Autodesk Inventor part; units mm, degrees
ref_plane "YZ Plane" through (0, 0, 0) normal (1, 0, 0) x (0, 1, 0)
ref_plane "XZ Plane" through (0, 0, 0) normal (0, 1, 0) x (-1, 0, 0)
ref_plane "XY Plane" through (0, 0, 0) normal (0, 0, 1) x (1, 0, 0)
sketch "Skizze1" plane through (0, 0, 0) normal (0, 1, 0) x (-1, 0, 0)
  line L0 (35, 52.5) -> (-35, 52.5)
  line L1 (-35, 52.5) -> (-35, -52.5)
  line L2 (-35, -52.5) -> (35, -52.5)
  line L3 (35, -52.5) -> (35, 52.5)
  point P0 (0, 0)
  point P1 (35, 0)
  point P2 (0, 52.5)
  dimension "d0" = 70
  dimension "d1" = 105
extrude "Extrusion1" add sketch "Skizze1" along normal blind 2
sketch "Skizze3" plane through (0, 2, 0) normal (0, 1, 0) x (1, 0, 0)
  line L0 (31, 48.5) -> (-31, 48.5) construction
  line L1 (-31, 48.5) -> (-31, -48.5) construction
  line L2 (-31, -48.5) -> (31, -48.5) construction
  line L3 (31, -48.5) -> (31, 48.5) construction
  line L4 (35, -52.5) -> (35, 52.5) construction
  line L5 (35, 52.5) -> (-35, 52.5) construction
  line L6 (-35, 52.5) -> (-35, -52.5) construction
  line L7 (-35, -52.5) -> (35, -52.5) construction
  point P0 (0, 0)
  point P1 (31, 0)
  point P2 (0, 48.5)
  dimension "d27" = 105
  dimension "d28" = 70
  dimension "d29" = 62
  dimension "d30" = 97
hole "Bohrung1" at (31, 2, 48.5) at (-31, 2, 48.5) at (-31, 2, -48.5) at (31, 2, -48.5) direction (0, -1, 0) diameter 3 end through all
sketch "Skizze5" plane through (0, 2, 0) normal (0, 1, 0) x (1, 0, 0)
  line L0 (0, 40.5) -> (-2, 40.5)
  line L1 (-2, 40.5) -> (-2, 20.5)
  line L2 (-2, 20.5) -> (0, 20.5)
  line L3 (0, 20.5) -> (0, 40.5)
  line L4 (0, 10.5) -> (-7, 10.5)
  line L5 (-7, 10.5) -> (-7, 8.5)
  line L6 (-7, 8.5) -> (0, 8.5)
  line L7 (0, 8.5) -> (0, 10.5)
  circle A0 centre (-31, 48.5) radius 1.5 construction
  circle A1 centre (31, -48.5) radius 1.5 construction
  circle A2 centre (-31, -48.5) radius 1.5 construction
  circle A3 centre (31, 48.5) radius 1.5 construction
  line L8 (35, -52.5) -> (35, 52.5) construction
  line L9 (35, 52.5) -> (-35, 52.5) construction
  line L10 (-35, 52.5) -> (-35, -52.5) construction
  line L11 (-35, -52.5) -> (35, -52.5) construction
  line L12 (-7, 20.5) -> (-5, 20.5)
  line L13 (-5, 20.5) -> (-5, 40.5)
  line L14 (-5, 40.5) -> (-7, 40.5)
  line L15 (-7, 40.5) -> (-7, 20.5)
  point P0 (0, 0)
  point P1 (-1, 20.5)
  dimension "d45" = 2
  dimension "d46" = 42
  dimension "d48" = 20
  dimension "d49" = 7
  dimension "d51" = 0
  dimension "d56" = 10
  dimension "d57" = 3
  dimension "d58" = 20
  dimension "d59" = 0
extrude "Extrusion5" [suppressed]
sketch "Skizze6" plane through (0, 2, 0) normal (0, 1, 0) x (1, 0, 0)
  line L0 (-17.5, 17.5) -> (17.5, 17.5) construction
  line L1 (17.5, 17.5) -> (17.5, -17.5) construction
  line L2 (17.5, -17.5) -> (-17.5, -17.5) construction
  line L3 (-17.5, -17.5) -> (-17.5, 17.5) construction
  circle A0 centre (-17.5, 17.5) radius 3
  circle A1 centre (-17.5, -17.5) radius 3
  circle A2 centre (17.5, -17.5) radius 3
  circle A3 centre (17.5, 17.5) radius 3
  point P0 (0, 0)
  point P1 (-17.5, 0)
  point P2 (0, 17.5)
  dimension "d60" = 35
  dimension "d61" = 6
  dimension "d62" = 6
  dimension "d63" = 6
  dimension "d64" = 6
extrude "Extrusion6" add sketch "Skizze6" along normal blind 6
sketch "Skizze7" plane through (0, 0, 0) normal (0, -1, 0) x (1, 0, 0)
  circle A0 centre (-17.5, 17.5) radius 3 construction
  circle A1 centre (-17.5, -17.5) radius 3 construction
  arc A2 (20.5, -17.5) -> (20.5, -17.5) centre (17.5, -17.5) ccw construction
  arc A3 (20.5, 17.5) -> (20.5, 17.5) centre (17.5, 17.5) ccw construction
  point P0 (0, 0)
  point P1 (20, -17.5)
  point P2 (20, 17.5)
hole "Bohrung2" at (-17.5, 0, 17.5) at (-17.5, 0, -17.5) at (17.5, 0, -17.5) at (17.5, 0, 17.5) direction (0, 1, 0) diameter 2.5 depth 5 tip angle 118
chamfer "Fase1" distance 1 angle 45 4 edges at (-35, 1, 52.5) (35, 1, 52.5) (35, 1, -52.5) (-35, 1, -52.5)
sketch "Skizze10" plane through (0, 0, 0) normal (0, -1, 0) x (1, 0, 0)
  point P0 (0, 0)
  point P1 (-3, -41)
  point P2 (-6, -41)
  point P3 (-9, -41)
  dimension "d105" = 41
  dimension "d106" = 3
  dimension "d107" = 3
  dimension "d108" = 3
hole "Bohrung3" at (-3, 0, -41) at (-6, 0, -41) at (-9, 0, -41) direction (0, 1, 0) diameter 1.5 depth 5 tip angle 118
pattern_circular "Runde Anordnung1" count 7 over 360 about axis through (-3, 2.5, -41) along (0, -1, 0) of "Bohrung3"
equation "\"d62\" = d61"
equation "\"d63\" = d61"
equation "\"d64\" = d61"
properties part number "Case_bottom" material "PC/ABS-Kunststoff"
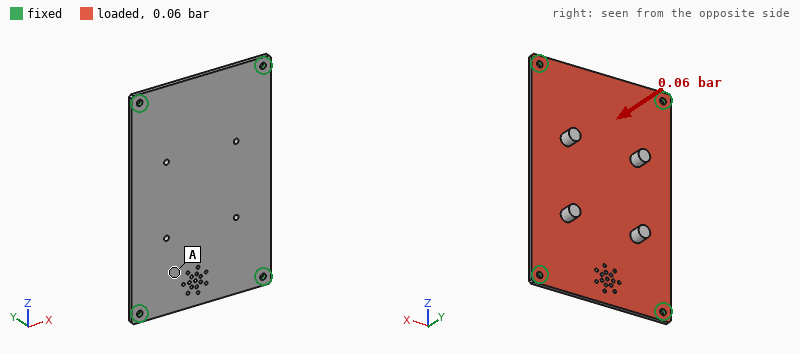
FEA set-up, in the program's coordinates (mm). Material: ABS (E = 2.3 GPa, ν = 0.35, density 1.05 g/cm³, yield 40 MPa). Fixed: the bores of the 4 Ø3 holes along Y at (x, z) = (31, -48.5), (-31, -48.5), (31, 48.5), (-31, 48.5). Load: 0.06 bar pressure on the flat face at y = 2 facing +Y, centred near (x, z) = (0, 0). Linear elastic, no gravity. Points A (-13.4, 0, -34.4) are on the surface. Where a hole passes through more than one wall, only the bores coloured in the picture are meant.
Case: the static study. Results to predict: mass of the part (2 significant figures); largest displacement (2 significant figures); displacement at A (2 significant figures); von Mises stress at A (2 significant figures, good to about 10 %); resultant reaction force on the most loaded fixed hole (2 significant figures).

16 g
1.4 mm
0.59 mm
1.5 MPa
11 N
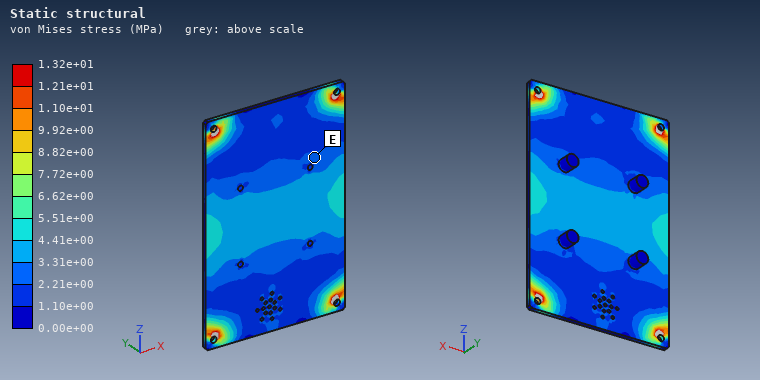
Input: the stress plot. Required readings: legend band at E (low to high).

2.21e+00 to 3.31e+00 MPa
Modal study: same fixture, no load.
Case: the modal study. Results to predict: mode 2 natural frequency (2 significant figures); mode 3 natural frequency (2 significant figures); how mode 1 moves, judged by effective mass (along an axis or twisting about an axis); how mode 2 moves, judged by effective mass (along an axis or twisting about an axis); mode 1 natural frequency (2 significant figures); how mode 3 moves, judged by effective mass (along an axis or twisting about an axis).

430 Hz
640 Hz
along Y
twisting about Z
250 Hz
twisting about X
